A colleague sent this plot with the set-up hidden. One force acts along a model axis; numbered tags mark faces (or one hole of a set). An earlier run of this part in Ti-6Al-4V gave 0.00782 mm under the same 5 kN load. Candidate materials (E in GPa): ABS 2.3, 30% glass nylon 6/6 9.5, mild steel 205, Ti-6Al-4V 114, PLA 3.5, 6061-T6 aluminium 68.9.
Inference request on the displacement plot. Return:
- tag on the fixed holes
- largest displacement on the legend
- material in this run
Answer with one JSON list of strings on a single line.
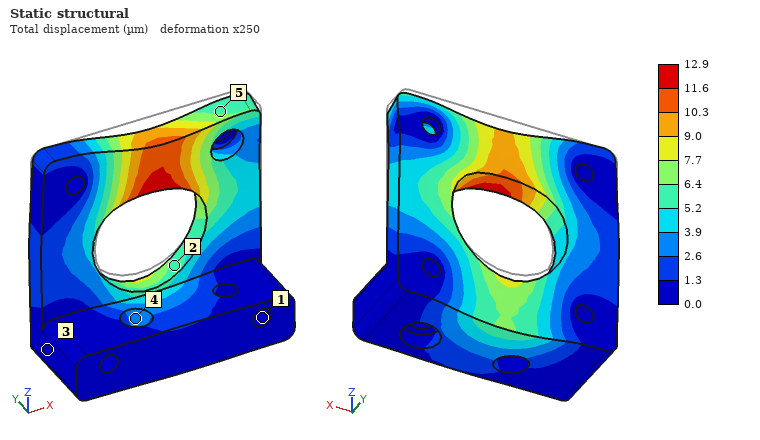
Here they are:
["1", "12.9 µm", "6061-T6 aluminium"]
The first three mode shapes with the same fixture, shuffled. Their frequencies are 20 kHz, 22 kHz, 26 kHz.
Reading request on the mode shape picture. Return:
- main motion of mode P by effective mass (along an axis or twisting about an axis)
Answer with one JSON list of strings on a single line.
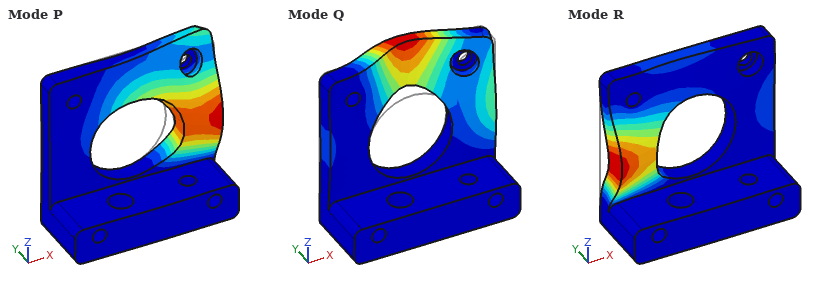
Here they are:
["along Y"]
